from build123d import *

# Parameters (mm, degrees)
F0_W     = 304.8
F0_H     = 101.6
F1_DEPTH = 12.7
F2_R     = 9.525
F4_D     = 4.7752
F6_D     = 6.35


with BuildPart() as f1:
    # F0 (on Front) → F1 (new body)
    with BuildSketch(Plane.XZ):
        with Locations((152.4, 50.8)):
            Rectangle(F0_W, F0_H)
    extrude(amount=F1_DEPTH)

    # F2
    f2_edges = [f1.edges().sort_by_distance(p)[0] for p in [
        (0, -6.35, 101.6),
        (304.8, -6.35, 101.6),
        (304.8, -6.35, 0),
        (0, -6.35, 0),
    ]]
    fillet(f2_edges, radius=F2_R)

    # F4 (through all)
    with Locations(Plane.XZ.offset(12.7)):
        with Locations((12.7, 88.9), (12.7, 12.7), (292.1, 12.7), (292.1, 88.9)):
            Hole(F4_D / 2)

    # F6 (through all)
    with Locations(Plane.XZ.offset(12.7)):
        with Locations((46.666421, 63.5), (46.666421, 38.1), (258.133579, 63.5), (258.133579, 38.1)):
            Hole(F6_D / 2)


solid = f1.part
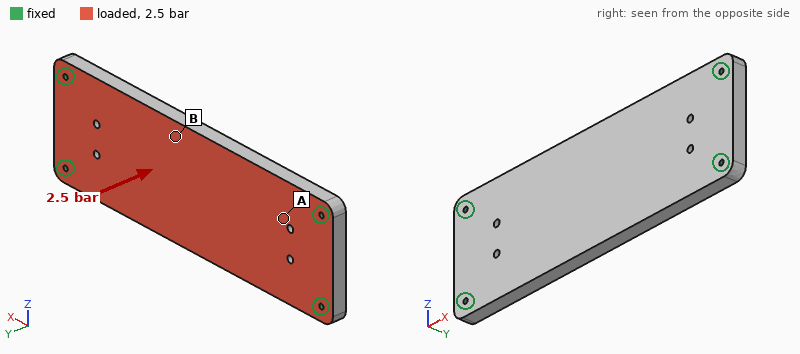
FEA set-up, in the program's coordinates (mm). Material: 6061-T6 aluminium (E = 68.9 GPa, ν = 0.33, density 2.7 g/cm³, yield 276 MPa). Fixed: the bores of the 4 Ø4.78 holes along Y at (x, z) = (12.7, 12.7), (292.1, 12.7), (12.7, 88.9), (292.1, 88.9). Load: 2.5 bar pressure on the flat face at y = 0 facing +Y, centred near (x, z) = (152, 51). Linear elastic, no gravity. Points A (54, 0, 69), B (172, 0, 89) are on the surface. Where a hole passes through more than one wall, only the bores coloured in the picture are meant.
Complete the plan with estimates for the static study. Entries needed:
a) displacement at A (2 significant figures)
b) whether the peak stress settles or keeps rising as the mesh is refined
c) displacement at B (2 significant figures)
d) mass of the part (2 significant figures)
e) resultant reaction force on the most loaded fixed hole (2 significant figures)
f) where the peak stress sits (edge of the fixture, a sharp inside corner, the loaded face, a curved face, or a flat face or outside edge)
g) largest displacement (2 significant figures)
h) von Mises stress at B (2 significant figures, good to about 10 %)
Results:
0.15 mm
keeps rising
0.44 mm
1.1 kg
1.9 kN
edge of the fixture
0.46 mm
34 MPa
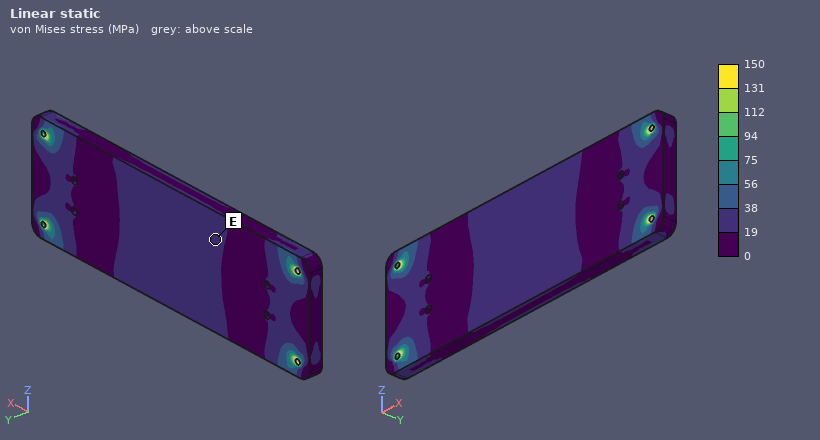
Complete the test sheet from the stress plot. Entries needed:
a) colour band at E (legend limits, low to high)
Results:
19 to 38 MPa
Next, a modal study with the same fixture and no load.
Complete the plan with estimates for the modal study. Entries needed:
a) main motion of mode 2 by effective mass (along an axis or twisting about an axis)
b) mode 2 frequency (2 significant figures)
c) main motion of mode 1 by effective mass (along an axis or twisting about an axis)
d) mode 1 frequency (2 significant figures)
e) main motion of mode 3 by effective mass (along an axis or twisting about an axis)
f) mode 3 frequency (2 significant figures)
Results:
twisting about X
1600 Hz
along Y
730 Hz
twisting about Z
2000 Hz
